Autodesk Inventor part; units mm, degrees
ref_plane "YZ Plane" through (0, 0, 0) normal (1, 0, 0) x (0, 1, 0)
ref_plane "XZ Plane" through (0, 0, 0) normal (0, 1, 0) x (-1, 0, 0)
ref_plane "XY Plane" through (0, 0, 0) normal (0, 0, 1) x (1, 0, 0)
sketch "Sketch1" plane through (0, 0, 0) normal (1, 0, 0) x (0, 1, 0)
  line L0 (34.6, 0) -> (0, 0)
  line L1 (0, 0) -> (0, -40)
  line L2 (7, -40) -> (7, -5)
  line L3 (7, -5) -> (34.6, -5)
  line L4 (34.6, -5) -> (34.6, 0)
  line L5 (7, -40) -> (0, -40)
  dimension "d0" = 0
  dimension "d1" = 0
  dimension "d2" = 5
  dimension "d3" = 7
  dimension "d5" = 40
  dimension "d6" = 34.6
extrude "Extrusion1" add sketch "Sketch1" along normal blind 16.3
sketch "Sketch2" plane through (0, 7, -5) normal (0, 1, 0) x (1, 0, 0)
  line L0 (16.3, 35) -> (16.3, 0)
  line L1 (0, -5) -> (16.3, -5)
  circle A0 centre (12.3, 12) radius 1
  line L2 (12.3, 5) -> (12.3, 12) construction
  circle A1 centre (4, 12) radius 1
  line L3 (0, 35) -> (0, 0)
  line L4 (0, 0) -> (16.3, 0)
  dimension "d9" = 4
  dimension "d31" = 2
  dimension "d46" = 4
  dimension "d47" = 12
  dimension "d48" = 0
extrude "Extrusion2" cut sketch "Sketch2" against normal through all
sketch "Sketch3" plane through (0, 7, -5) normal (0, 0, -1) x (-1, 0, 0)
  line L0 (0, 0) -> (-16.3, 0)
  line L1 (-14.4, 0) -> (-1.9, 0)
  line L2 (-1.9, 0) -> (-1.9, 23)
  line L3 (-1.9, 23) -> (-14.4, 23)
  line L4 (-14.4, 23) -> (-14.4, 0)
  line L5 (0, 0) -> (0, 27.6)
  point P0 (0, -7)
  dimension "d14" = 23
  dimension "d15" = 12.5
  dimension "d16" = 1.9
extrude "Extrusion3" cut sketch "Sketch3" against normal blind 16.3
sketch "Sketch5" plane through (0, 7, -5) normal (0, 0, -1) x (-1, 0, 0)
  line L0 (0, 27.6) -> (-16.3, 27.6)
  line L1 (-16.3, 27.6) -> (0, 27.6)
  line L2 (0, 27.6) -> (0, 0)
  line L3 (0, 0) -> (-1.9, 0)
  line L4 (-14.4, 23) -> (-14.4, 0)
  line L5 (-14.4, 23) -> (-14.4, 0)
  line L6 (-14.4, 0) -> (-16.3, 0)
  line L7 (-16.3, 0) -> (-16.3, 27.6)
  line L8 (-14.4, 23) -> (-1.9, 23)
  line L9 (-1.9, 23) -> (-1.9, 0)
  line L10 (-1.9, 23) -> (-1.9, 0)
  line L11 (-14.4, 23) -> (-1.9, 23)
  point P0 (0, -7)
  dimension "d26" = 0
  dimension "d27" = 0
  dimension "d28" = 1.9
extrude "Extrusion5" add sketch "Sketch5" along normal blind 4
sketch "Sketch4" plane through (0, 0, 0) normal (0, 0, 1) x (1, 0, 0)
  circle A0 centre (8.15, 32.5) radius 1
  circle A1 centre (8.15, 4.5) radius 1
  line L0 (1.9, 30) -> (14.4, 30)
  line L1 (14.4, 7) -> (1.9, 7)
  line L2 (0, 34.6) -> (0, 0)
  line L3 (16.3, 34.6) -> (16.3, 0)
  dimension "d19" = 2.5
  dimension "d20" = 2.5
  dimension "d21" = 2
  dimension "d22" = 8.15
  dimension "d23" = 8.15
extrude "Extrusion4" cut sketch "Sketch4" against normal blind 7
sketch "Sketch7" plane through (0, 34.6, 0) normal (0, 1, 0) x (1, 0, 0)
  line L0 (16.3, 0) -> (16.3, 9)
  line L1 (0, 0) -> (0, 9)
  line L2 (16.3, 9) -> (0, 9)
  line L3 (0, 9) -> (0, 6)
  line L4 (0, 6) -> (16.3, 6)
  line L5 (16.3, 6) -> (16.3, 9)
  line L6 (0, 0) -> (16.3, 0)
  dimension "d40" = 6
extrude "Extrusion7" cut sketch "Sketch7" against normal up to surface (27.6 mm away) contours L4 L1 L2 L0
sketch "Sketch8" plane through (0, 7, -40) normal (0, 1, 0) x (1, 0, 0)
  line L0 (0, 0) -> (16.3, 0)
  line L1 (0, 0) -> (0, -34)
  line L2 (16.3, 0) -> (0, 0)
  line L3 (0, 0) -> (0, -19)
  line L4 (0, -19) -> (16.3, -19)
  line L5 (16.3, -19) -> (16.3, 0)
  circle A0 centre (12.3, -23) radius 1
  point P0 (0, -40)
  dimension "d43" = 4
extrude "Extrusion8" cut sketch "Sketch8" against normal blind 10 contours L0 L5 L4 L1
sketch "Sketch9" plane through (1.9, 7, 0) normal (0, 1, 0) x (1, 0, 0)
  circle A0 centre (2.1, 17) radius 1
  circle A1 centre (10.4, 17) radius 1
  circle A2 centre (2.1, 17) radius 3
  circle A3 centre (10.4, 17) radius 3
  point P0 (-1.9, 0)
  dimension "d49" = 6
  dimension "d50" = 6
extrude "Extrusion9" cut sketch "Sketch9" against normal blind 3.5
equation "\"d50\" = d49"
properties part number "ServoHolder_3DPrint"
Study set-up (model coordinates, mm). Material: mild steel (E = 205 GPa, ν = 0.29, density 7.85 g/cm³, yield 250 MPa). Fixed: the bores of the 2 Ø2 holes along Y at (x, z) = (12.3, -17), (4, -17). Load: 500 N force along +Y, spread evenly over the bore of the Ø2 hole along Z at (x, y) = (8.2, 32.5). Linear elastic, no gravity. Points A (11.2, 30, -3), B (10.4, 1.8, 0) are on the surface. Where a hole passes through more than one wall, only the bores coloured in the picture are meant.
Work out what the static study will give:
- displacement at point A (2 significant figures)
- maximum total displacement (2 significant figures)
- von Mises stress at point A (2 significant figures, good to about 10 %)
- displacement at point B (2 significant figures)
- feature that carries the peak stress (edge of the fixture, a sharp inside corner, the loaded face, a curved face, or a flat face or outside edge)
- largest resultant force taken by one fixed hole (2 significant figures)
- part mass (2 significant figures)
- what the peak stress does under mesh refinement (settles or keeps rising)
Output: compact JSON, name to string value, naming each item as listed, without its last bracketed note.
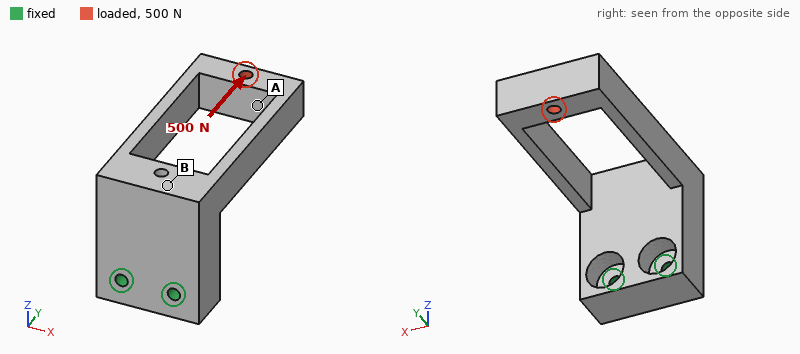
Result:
{"displacement at point A": "49 µm", "maximum total displacement": "58 µm", "von Mises stress at point A": "46 MPa", "displacement at point B": "23 µm", "feature that carries the peak stress": "edge of the fixture", "largest resultant force taken by one fixed hole": "250 N", "part mass": "24 g", "what the peak stress does under mesh refinement": "keeps rising"}
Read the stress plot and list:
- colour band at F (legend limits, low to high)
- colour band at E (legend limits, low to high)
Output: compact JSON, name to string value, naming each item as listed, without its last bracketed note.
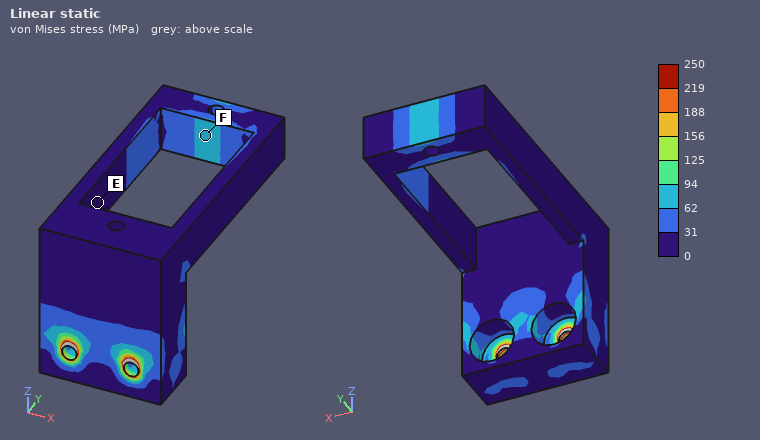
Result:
{"colour band at F": "62 to 94 MPa", "colour band at E": "0 to 31 MPa"}
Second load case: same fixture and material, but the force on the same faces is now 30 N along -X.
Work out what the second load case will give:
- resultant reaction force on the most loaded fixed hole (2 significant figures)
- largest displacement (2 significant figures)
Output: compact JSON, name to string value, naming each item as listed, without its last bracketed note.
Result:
{"resultant reaction force on the most loaded fixed hole": "97 N", "largest displacement": "33 µm"}
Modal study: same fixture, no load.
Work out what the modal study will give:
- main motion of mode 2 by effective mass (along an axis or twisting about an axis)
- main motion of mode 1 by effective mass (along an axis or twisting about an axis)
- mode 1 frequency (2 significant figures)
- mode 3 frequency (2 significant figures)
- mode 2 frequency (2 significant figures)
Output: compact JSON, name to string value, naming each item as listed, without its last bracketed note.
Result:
{"main motion of mode 2 by effective mass": "along Z", "main motion of mode 1 by effective mass": "along X", "mode 1 frequency": "2200 Hz", "mode 3 frequency": "7300 Hz", "mode 2 frequency": "2700 Hz"}
